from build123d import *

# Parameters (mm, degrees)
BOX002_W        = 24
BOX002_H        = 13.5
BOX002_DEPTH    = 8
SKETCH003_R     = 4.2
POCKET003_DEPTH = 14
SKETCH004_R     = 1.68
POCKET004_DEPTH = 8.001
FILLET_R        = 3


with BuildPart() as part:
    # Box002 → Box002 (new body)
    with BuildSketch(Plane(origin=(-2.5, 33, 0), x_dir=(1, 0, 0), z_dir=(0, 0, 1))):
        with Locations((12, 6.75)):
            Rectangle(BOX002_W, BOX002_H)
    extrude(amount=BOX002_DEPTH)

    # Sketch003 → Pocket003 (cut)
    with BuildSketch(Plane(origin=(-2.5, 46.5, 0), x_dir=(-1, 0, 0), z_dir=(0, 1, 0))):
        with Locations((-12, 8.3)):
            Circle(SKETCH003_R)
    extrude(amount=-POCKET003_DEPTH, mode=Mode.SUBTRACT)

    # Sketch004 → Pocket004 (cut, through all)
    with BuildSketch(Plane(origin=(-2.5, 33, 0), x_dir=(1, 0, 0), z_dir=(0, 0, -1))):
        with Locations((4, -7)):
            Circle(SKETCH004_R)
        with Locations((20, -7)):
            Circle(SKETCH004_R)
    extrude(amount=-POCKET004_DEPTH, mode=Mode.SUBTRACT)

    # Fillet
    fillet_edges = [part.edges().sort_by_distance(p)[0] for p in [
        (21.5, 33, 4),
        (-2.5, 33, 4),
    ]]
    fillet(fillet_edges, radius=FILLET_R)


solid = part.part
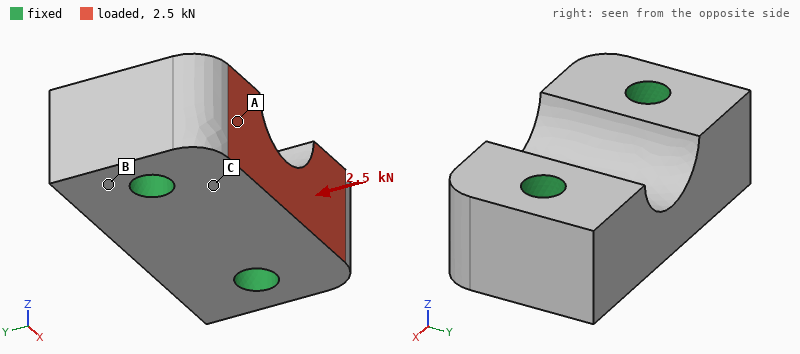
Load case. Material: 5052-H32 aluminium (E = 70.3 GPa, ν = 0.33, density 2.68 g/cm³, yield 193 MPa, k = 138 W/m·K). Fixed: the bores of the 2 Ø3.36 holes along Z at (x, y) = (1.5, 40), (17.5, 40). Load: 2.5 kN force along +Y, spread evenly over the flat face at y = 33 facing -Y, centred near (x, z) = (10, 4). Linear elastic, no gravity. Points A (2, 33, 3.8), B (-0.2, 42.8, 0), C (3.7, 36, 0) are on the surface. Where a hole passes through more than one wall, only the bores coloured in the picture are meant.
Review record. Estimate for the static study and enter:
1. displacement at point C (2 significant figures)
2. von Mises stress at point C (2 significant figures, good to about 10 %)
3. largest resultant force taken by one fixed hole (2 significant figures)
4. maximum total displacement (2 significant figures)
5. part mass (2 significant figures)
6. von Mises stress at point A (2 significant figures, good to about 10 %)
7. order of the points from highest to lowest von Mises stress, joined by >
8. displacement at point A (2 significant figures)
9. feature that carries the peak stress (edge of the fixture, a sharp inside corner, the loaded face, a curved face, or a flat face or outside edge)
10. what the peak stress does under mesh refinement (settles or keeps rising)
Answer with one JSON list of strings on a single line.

["1.8 µm", "27 MPa", "1.3 kN", "4.4 µm", "5.6 g", "17 MPa", "C > A > B", "2.1 µm", "edge of the fixture", "keeps rising"]
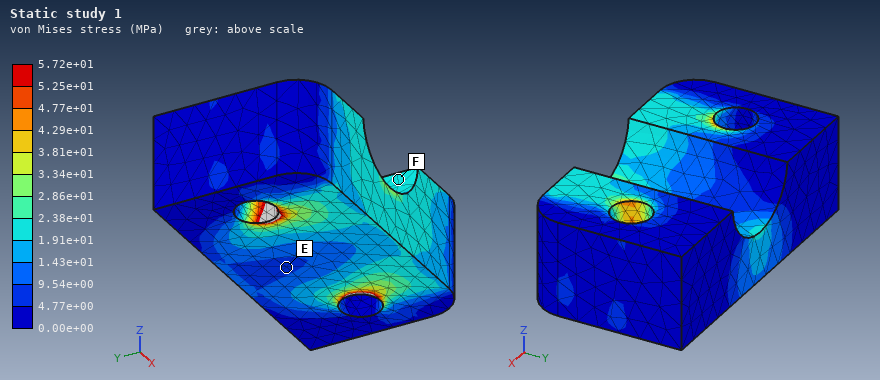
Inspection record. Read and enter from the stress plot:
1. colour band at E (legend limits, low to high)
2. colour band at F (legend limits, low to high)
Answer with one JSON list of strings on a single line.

["4.77e+00 to 9.54e+00 MPa", "1.91e+01 to 2.38e+01 MPa"]
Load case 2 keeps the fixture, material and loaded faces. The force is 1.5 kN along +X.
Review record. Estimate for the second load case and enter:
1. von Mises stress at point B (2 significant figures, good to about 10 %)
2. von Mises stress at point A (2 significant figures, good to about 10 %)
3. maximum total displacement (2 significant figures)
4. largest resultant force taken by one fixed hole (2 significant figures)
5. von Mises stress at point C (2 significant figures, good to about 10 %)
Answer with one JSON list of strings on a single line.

["6.4 MPa", "23 MPa", "4.8 µm", "880 N", "21 MPa"]
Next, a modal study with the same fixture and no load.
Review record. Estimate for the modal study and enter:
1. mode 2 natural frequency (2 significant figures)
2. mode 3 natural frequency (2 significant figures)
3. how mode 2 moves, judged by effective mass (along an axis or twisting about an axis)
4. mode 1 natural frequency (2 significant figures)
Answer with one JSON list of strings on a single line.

["80 kHz", "88 kHz", "along Z", "72 kHz"]
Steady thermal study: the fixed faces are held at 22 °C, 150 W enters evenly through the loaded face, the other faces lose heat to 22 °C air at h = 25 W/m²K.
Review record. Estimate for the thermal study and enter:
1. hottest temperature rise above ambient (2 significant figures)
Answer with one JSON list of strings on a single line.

["63 K"]
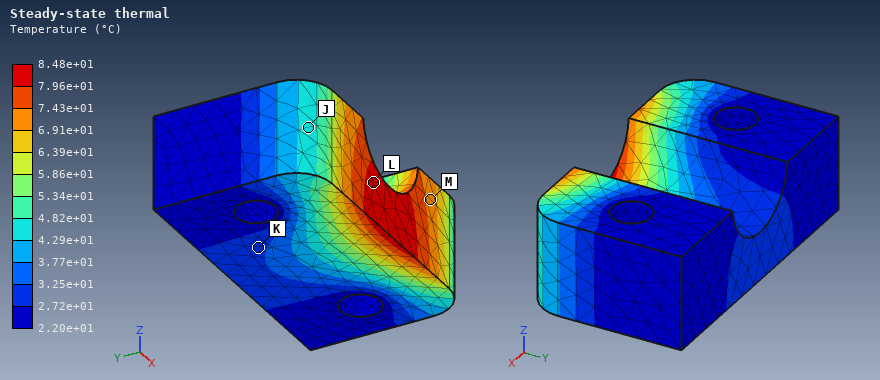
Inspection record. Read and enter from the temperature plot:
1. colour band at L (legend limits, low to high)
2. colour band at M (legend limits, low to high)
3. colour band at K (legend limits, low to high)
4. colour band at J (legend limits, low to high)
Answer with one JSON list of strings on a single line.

["7.96e+01 to 8.48e+01 °C", "6.91e+01 to 7.43e+01 °C", "2.72e+01 to 3.25e+01 °C", "4.29e+01 to 4.82e+01 °C"]
